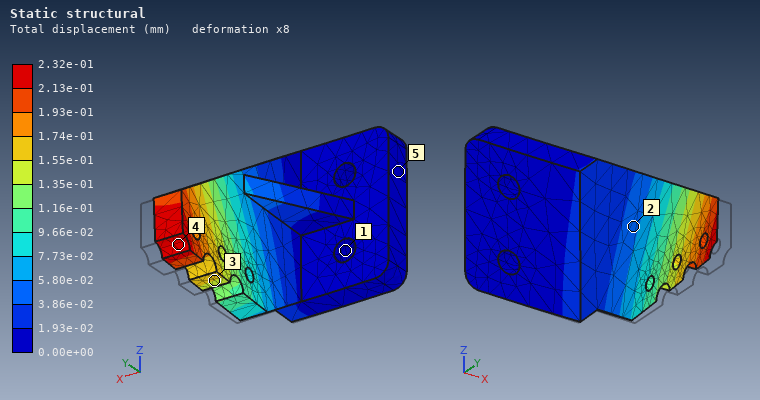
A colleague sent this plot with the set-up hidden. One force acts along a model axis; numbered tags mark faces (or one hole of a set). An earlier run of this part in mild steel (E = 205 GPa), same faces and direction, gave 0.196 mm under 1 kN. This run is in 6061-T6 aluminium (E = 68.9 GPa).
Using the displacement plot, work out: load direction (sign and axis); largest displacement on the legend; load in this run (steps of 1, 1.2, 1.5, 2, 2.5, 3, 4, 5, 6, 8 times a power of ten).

-X
2.32e-01 mm
400 N
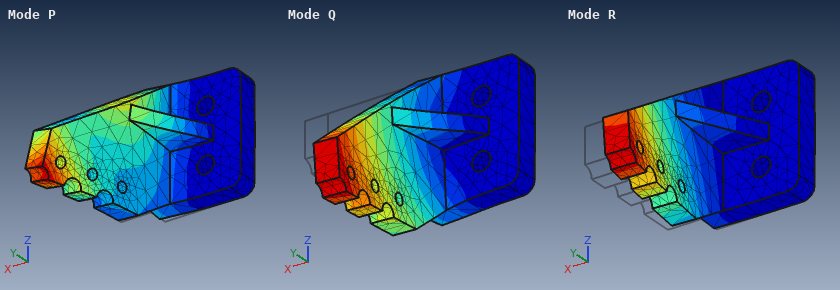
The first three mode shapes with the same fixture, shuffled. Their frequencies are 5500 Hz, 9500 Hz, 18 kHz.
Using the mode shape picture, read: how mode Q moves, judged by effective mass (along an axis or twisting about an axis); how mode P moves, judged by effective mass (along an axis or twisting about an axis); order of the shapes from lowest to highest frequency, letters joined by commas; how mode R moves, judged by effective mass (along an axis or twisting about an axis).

along Z
along Y
R, Q, P
along X
